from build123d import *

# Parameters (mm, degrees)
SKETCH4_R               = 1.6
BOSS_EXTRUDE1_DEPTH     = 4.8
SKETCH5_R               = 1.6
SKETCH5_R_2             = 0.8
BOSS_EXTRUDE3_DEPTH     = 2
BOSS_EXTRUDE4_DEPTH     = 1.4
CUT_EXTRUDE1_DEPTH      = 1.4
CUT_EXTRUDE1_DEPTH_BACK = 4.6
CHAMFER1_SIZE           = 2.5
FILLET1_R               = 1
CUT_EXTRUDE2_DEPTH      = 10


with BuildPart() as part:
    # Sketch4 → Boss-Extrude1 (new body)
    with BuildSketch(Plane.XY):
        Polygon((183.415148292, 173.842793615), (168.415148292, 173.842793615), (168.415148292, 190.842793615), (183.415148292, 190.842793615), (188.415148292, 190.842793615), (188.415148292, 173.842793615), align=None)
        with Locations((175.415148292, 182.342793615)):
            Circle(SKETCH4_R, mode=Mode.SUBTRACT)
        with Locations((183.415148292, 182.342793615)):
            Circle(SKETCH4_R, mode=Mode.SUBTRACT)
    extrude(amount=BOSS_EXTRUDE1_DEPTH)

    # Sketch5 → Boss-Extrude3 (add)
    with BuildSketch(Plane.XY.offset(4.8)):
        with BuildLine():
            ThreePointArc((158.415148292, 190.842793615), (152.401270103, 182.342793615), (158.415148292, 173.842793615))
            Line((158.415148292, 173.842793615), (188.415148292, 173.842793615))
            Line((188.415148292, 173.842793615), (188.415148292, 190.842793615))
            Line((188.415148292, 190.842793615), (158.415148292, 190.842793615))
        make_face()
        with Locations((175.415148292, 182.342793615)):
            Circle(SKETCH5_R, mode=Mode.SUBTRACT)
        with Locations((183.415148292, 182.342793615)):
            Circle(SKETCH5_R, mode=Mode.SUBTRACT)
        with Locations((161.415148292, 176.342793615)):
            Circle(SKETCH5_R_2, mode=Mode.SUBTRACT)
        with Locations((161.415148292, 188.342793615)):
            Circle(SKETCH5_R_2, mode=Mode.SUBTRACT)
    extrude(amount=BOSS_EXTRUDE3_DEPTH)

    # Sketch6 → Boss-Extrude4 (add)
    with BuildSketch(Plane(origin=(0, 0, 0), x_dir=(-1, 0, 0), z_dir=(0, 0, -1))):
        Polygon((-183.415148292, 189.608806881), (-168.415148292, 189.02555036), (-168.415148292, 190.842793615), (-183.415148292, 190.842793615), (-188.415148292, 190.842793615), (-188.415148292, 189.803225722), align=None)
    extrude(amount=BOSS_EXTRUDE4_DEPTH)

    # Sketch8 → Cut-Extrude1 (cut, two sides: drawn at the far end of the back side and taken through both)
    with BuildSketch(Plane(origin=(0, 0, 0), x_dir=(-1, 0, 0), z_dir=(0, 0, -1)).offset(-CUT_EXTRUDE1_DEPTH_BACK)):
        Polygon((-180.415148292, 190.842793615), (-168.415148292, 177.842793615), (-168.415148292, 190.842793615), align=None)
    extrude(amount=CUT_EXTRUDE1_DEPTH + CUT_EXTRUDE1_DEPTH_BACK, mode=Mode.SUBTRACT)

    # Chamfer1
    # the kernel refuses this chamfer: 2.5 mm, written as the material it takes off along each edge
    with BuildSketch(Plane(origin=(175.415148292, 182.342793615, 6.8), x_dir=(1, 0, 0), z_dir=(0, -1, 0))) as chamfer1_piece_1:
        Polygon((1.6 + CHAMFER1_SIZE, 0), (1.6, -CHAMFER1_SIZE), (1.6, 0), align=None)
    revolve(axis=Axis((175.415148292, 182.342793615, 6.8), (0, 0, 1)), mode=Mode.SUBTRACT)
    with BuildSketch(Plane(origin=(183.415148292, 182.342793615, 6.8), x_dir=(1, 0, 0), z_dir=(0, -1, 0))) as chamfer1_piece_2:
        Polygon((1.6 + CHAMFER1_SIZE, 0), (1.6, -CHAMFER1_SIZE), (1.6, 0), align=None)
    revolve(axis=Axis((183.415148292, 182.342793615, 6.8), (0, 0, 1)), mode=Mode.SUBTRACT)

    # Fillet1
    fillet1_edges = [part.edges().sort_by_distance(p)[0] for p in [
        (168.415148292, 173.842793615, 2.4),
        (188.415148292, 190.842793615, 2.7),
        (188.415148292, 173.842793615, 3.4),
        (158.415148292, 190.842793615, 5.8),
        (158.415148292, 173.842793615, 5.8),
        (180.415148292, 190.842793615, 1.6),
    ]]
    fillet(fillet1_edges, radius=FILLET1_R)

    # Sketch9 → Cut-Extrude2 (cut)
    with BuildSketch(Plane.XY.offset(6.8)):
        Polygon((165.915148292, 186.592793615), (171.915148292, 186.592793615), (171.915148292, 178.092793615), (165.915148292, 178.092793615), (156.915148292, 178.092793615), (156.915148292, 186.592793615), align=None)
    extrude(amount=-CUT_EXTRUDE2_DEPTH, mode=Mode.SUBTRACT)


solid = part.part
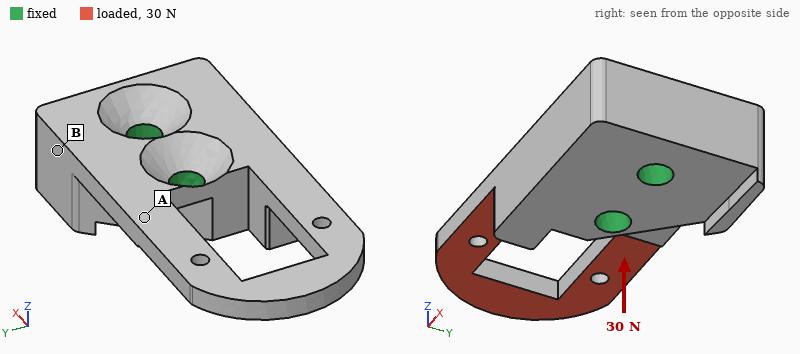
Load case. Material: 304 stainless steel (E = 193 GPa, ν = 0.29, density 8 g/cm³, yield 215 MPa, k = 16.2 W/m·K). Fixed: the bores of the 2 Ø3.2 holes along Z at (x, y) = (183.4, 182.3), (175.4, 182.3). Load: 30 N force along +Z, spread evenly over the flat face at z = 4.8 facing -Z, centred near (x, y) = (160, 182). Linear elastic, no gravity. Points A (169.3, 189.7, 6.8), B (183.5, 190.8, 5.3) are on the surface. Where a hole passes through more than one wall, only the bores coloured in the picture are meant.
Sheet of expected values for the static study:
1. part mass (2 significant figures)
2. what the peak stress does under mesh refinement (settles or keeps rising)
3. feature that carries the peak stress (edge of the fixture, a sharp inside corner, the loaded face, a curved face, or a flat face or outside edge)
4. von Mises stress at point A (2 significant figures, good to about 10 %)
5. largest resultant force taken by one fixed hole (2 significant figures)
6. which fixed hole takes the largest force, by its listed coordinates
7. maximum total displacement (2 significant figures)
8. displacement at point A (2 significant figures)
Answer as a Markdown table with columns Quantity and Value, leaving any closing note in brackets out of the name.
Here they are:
| Quantity | Value |
|---|---|
| part mass | 16 g |
| what the peak stress does under mesh refinement | keeps rising |
| feature that carries the peak stress | a sharp inside corner |
| von Mises stress at point A | 30 MPa |
| largest resultant force taken by one fixed hole | 70 N |
| which fixed hole takes the largest force, by its listed coordinates | (175.4, 182.3) |
| maximum total displacement | 37 µm |
| displacement at point A | 7.0 µm |
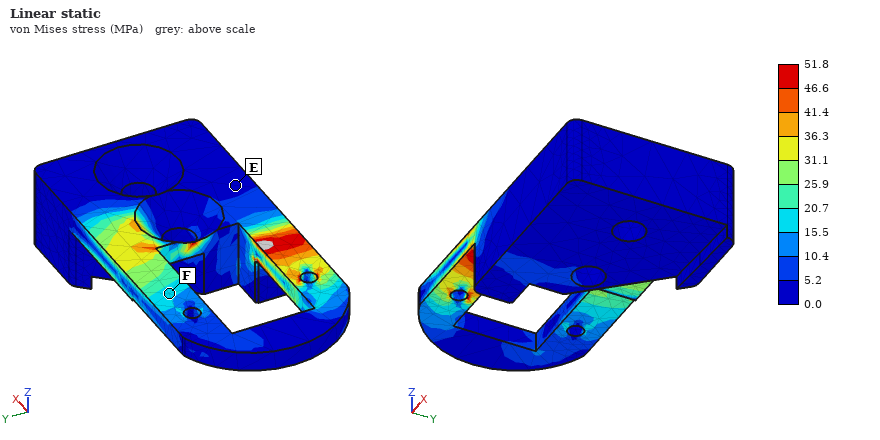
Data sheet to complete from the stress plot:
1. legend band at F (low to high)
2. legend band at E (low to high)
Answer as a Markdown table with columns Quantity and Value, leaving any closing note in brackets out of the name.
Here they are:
| Quantity | Value |
|---|---|
| legend band at F | 15.5 to 20.7 MPa |
| legend band at E | 0.0 to 5.2 MPa |
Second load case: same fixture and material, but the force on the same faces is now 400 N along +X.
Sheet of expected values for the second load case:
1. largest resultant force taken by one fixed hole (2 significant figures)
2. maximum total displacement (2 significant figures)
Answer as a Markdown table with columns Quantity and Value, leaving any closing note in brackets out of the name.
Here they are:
| Quantity | Value |
|---|---|
| largest resultant force taken by one fixed hole | 220 N |
| maximum total displacement | 53 µm |
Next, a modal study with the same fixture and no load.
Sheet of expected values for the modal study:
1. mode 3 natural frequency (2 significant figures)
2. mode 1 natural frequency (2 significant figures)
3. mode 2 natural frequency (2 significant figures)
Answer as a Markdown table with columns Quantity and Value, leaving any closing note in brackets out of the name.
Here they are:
| Quantity | Value |
|---|---|
| mode 3 natural frequency | 10 kHz |
| mode 1 natural frequency | 3600 Hz |
| mode 2 natural frequency | 9100 Hz |
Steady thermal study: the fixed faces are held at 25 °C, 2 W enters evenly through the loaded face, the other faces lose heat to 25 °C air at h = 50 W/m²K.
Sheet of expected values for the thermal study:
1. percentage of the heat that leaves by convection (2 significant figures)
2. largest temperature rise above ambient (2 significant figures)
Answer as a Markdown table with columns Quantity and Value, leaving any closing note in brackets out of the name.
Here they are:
| Quantity | Value |
|---|---|
| percentage of the heat that leaves by convection | 47 % |
| largest temperature rise above ambient | 64 K |
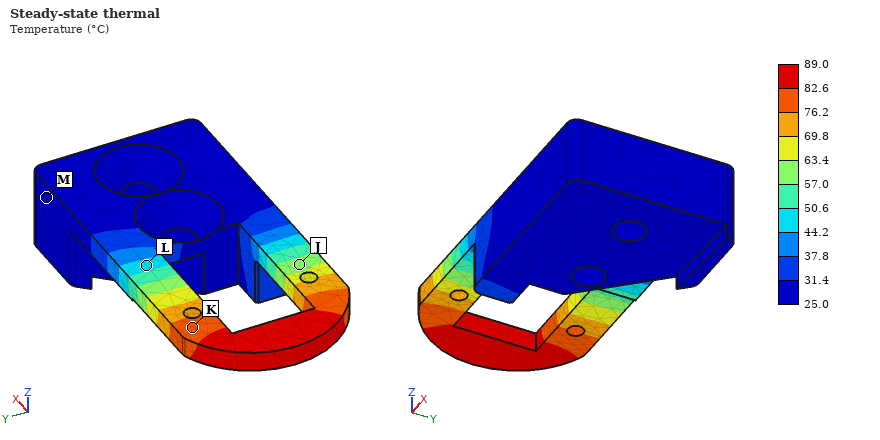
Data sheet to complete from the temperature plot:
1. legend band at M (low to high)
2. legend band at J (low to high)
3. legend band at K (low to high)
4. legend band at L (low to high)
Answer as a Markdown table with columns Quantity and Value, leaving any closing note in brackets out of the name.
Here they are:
| Quantity | Value |
|---|---|
| legend band at M | 25.0 to 31.4 °C |
| legend band at J | 57.0 to 63.4 °C |
| legend band at K | 76.2 to 82.6 °C |
| legend band at L | 44.2 to 50.6 °C |
